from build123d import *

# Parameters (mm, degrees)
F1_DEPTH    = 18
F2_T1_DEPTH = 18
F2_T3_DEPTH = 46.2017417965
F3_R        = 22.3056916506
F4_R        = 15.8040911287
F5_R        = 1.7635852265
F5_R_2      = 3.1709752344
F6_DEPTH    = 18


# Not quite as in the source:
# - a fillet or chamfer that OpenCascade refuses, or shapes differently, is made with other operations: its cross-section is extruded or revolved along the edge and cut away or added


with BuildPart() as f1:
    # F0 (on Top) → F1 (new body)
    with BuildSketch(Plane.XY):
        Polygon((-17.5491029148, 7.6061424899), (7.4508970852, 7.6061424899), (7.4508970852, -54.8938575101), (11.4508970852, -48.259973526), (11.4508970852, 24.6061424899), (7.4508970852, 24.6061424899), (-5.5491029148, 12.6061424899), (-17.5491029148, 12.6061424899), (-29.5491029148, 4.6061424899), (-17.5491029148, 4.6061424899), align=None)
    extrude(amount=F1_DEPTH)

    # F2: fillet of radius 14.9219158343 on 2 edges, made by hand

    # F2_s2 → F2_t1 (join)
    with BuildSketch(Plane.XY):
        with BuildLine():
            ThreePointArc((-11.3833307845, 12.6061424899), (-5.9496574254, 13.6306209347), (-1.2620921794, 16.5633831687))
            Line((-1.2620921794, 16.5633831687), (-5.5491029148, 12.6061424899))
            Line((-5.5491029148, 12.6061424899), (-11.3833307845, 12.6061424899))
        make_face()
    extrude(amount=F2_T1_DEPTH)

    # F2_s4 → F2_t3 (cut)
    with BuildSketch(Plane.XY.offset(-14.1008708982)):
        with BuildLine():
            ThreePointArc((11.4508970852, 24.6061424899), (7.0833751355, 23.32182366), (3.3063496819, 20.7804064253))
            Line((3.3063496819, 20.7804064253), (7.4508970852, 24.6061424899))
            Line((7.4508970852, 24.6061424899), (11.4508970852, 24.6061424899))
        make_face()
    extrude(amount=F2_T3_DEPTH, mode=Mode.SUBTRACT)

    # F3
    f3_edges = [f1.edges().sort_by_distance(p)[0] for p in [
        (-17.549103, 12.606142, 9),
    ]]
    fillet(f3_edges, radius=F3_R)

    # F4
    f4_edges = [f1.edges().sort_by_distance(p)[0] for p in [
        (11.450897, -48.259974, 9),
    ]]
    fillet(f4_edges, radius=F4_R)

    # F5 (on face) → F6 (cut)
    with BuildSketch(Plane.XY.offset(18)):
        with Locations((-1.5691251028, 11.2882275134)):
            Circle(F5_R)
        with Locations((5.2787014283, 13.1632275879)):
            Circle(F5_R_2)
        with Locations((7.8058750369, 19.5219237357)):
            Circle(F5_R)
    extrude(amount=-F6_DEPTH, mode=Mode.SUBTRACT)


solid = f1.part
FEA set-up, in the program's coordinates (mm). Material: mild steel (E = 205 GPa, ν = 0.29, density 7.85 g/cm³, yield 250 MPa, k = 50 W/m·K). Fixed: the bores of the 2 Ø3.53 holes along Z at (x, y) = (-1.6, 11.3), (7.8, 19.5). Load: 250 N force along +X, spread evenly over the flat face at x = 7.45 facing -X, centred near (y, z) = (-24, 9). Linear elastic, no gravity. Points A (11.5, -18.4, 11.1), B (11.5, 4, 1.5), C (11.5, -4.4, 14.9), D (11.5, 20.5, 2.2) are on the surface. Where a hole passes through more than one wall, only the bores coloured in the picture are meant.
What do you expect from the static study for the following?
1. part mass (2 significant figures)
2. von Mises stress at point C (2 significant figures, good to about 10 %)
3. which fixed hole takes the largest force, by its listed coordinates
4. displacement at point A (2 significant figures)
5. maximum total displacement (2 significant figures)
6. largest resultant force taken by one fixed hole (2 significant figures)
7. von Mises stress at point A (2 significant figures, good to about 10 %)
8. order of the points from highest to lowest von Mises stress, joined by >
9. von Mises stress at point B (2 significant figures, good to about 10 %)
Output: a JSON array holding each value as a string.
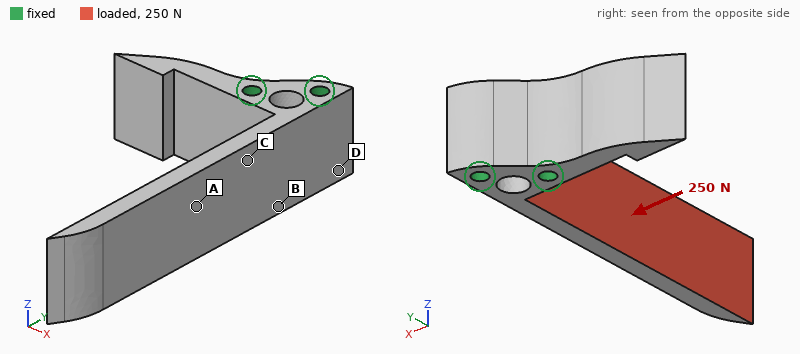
["71 g", "110 MPa", "(-1.6, 11.3)", "0.13 mm", "0.46 mm", "1.1 kN", "56 MPa", "B > C > A > D", "140 MPa"]
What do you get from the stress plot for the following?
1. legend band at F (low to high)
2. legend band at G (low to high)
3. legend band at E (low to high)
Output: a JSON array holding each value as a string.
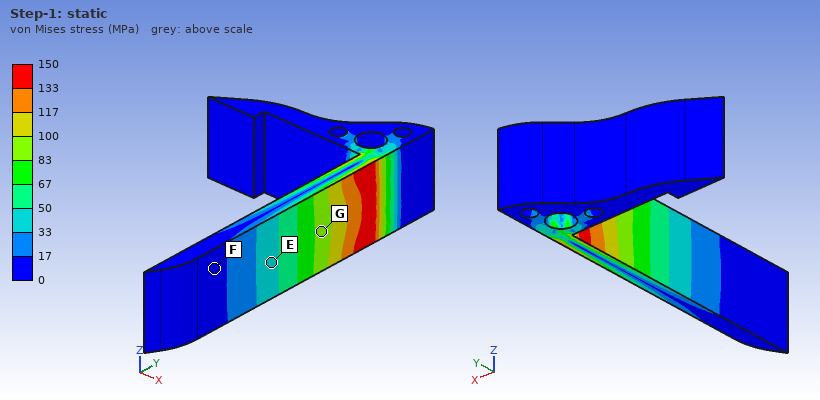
["0 to 17 MPa", "83 to 100 MPa", "33 to 50 MPa"]
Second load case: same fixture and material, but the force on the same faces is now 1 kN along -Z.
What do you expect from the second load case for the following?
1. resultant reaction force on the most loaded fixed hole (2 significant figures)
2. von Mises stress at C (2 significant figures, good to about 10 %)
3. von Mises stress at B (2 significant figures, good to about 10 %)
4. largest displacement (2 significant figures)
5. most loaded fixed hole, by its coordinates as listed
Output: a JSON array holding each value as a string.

["1.3 kN", "62 MPa", "110 MPa", "0.15 mm", "(-1.6, 11.3)"]
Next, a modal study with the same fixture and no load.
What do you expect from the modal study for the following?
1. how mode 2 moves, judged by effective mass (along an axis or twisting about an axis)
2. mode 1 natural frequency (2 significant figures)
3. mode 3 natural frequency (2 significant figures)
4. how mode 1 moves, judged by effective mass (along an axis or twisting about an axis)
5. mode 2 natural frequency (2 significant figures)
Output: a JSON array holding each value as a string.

["along Z", "870 Hz", "5300 Hz", "along X", "3000 Hz"]
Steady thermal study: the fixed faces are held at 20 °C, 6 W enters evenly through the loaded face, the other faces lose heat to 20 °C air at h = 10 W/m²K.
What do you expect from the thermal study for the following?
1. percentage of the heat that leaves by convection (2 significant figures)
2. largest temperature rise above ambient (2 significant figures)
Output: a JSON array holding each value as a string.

["11 %", "56 K"]
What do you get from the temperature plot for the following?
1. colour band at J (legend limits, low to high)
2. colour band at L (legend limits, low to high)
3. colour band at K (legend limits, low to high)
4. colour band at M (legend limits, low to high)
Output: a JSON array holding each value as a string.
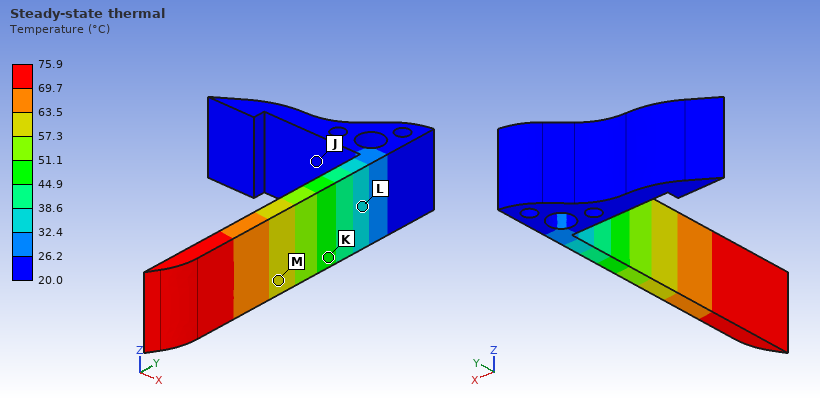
["20.0 to 26.2 °C", "32.4 to 38.6 °C", "44.9 to 51.1 °C", "57.3 to 63.5 °C"]
